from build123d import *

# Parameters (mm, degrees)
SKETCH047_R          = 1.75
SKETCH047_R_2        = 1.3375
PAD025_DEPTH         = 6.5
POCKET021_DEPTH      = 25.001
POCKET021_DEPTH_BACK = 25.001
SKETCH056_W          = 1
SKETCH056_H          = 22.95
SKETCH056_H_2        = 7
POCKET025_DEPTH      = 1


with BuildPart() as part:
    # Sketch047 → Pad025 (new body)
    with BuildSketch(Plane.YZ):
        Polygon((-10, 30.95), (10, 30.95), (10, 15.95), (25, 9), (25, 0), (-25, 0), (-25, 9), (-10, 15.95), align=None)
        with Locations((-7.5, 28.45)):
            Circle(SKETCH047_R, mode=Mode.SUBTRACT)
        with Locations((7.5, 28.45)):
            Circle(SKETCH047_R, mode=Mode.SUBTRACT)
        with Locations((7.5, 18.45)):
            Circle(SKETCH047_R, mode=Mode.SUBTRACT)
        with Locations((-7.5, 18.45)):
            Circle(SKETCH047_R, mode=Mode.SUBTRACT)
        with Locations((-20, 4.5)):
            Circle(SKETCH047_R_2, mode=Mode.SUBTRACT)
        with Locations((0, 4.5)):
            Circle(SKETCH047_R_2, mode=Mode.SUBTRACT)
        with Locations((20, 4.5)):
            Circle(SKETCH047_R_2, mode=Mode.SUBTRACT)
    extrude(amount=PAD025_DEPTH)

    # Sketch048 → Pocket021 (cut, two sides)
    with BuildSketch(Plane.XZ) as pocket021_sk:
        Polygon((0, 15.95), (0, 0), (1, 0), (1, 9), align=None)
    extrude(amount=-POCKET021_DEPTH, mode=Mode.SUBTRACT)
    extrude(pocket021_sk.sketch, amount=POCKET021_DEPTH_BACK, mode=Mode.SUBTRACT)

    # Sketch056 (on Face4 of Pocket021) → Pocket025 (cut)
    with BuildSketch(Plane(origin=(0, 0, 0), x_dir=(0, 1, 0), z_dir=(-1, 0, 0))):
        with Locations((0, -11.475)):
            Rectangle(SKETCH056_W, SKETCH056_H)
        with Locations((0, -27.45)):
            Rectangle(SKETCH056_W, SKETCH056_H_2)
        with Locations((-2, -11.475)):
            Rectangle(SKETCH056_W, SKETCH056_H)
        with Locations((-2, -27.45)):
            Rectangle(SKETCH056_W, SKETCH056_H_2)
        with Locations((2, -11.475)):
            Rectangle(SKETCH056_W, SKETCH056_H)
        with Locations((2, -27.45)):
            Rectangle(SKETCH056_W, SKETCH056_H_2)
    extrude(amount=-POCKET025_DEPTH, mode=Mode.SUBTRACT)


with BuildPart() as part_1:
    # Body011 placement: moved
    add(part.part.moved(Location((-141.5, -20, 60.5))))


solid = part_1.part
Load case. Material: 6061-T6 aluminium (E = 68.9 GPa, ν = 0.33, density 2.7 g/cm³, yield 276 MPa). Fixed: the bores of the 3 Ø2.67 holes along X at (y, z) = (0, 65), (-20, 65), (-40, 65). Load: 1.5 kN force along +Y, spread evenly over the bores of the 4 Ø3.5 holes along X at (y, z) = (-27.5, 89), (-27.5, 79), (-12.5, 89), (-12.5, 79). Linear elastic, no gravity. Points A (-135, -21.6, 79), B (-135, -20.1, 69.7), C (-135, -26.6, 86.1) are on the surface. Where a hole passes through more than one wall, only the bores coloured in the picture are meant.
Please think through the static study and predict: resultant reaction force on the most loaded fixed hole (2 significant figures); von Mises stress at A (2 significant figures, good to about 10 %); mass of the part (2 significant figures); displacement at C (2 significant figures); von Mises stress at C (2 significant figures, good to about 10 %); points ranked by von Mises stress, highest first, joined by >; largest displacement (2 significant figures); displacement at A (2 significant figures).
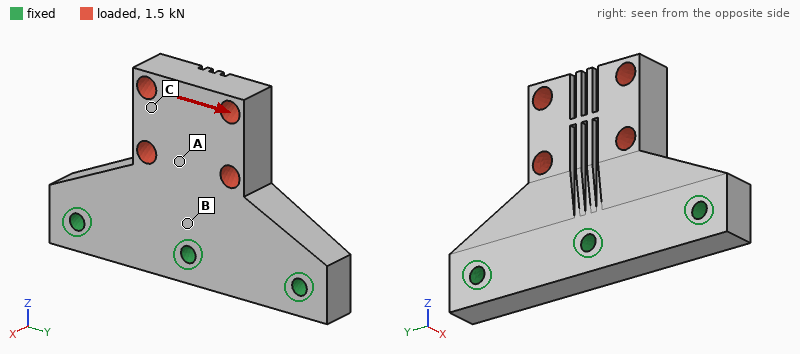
920 N
25 MPa
15 g
18 µm
18 MPa
A > C > B
25 µm
8.4 µm
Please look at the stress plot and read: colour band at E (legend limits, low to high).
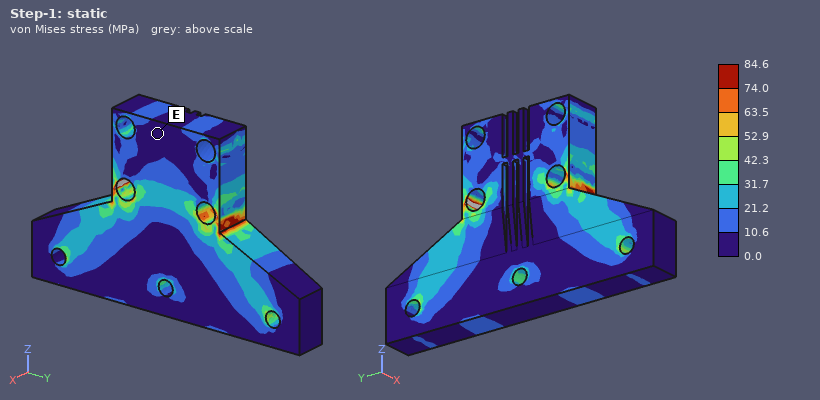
0.0 to 10.6 MPa
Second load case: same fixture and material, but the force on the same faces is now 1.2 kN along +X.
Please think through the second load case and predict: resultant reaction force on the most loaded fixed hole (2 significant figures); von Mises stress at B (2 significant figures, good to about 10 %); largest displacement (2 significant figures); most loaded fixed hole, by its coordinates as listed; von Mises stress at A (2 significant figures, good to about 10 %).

950 N
140 MPa
0.20 mm
(-20, 65)
53 MPa
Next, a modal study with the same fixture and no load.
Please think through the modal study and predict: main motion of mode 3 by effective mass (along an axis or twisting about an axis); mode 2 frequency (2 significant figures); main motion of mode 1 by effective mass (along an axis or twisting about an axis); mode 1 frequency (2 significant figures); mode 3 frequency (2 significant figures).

along Y
19 kHz
along X
6700 Hz
21 kHz
